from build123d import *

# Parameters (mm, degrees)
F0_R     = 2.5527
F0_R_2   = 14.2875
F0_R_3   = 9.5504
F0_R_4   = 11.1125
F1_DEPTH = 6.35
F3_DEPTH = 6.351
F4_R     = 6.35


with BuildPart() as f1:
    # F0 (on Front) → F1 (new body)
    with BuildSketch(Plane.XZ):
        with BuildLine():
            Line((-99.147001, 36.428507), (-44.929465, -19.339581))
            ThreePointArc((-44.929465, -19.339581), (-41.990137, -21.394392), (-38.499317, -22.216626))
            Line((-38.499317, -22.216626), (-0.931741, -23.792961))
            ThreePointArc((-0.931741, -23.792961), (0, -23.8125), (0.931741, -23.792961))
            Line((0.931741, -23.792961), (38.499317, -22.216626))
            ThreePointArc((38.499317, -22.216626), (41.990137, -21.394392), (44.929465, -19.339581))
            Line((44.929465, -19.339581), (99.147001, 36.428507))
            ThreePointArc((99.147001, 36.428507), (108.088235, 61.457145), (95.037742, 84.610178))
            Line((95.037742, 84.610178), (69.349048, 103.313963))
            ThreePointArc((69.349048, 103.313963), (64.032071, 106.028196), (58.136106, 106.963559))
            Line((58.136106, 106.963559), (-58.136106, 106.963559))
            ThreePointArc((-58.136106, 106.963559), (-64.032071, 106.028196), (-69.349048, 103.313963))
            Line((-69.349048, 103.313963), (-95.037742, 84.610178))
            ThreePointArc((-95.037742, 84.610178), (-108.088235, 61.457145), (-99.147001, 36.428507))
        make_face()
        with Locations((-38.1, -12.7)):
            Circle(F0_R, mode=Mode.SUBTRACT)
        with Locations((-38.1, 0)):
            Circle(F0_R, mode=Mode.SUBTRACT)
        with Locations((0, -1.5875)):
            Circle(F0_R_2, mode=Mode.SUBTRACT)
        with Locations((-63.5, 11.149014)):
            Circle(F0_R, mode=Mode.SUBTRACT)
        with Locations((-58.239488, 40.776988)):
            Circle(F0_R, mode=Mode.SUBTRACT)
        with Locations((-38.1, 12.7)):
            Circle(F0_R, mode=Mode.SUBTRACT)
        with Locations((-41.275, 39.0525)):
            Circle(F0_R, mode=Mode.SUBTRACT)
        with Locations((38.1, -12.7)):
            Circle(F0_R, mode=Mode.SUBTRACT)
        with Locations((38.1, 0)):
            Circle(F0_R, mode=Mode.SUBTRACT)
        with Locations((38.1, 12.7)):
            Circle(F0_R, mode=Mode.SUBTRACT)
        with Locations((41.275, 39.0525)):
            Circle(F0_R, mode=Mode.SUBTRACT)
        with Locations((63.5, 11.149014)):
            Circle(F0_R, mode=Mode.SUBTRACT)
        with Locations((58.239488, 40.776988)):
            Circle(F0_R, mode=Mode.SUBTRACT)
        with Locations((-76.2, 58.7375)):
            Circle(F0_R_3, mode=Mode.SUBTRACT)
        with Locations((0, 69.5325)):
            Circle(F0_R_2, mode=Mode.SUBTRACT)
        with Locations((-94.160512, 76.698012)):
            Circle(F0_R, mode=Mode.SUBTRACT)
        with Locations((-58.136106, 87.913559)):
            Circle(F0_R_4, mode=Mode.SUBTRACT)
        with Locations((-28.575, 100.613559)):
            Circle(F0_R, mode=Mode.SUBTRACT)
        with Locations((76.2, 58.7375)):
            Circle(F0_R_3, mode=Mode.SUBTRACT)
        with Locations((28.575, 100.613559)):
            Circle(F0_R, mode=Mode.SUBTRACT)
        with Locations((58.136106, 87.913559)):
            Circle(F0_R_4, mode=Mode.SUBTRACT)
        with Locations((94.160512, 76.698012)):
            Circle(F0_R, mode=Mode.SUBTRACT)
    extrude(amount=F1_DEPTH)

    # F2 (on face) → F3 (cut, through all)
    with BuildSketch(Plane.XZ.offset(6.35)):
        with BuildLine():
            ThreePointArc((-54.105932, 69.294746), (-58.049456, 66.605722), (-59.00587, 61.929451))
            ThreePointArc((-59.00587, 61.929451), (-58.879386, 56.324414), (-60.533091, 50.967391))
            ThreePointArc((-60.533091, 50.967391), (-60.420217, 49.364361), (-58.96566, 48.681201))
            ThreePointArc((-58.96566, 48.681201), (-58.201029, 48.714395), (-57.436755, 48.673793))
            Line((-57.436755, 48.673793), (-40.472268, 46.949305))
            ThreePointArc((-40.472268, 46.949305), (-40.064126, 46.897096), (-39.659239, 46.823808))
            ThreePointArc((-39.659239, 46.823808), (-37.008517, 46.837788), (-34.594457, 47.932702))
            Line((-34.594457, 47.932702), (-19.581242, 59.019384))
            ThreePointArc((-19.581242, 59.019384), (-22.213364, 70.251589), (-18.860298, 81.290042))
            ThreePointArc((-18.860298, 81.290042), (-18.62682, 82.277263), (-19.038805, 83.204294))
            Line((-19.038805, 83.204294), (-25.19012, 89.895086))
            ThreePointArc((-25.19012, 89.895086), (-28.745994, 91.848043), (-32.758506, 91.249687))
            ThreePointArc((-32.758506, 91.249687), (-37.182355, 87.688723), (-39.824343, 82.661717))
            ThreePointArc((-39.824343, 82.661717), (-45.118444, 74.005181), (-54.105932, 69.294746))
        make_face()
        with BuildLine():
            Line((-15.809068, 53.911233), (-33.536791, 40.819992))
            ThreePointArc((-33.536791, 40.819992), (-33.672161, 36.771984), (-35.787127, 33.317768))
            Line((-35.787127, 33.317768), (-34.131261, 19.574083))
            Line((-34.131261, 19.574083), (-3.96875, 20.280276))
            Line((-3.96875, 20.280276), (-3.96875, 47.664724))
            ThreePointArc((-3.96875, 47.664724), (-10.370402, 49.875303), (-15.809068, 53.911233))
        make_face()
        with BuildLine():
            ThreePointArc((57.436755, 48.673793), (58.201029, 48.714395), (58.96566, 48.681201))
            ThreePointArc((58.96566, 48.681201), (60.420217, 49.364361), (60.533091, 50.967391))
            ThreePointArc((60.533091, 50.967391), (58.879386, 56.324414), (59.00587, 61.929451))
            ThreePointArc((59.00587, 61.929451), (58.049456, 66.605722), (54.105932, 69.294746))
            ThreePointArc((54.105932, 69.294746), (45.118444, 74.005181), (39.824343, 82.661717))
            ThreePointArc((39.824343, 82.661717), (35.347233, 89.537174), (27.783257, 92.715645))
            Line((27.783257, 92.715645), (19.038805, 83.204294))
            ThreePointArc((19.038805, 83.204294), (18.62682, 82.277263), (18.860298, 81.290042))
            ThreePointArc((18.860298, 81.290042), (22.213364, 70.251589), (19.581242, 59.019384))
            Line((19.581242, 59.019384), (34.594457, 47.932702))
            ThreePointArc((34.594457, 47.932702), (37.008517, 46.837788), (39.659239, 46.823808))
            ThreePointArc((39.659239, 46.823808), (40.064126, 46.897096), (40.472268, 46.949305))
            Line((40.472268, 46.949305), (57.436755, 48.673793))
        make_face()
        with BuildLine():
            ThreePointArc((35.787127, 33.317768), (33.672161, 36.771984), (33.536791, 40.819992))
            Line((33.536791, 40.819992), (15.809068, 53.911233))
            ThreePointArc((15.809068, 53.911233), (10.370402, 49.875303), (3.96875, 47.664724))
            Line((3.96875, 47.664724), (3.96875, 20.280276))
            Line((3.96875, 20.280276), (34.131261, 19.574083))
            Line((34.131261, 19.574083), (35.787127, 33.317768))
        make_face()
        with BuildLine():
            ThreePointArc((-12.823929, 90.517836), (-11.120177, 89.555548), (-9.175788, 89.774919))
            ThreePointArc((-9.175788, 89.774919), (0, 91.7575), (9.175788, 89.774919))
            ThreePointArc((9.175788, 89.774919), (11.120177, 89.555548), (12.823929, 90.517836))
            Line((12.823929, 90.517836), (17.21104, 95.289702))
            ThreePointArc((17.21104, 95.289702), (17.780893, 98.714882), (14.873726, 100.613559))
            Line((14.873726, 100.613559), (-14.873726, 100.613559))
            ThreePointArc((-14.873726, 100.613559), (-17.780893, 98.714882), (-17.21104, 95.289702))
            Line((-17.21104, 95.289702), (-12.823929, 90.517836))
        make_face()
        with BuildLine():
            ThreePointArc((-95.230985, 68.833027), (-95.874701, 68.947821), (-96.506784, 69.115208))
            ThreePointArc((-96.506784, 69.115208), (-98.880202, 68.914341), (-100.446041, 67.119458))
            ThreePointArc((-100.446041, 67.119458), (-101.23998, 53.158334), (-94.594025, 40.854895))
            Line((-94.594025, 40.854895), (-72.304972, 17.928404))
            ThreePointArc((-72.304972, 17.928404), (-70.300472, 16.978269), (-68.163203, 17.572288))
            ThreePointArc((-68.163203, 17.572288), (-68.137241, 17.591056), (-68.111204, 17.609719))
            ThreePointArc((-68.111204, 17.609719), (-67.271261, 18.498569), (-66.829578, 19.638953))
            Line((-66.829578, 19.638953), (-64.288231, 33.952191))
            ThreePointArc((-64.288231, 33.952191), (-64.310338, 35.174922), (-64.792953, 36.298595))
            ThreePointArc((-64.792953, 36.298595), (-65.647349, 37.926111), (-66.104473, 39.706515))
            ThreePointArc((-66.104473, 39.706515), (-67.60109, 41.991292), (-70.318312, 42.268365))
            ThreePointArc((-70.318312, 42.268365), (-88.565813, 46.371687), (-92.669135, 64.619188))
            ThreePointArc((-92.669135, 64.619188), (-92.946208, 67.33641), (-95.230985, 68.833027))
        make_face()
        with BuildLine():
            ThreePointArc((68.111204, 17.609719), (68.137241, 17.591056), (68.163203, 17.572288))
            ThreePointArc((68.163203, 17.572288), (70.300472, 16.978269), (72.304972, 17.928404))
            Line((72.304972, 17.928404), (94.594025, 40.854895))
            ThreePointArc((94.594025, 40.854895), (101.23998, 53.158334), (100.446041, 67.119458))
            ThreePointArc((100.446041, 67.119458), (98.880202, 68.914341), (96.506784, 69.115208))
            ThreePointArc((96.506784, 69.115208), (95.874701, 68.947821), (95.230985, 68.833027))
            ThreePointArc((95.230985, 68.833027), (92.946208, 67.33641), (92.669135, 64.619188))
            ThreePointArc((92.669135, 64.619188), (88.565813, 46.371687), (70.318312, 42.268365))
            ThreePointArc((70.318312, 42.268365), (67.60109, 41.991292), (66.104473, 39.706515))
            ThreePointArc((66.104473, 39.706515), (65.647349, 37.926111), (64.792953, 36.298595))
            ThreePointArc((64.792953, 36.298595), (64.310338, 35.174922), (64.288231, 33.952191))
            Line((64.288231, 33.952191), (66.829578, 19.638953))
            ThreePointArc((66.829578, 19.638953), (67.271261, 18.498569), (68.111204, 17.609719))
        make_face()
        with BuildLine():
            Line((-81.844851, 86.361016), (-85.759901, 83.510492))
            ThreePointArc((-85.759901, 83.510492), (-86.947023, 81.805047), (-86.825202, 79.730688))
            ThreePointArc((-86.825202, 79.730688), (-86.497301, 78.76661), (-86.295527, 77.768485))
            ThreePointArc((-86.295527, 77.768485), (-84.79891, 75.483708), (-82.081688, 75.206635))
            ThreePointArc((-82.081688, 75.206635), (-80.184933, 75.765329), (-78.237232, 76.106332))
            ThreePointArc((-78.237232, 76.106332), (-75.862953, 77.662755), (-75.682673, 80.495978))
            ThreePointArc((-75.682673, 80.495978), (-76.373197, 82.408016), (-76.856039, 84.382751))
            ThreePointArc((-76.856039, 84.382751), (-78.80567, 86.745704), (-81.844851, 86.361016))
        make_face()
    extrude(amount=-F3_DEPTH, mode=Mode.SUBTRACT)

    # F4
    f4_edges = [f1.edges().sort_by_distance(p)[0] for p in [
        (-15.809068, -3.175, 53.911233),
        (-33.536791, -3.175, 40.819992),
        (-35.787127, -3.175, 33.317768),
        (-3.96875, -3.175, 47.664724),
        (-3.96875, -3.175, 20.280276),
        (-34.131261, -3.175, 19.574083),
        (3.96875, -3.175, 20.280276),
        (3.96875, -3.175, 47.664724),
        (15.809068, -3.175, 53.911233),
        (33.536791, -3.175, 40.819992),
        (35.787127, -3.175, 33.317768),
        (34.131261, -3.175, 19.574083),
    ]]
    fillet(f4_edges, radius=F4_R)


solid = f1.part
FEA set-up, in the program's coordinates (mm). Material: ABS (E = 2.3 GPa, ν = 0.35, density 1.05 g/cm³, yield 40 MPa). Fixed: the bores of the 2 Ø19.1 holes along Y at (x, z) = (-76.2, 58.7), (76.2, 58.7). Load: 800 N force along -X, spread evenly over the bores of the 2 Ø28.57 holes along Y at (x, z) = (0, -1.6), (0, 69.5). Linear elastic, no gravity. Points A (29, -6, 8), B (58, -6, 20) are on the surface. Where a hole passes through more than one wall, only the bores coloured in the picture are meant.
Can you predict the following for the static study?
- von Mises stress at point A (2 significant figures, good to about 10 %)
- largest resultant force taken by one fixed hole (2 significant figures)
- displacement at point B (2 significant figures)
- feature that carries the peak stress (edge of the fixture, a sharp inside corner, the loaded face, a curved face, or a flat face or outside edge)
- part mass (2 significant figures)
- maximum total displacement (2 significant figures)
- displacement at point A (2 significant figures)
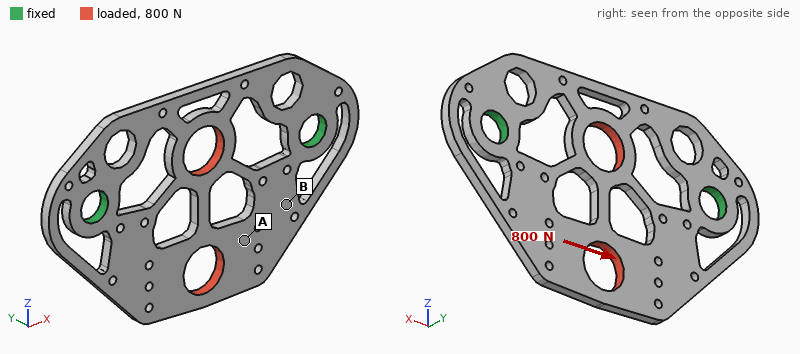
1.7 MPa
420 N
0.15 mm
a curved face
88 g
0.26 mm
0.20 mm
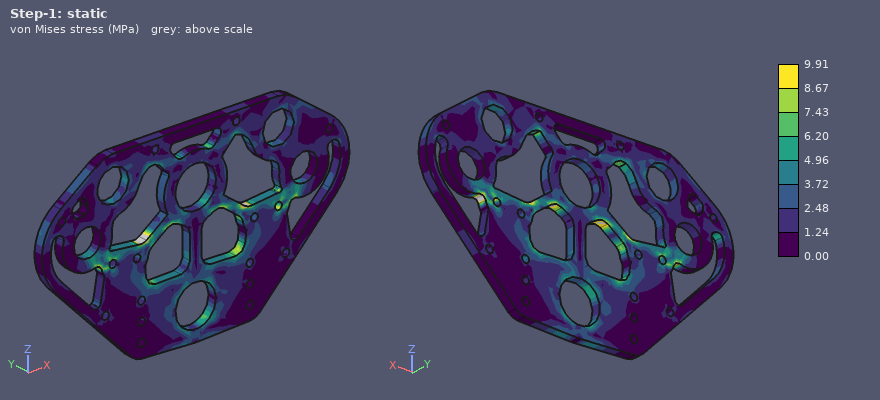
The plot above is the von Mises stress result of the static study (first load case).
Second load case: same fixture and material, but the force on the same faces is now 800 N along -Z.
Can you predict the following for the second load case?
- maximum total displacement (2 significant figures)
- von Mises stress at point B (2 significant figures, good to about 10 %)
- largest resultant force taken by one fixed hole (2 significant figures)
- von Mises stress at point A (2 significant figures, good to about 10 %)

0.22 mm
2.0 MPa
410 N
1.5 MPa
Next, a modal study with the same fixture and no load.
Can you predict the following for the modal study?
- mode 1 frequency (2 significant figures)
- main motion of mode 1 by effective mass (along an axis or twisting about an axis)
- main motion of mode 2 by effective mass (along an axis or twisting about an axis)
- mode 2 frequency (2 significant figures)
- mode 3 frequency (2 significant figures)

150 Hz
along Y
along Y
350 Hz
390 Hz
